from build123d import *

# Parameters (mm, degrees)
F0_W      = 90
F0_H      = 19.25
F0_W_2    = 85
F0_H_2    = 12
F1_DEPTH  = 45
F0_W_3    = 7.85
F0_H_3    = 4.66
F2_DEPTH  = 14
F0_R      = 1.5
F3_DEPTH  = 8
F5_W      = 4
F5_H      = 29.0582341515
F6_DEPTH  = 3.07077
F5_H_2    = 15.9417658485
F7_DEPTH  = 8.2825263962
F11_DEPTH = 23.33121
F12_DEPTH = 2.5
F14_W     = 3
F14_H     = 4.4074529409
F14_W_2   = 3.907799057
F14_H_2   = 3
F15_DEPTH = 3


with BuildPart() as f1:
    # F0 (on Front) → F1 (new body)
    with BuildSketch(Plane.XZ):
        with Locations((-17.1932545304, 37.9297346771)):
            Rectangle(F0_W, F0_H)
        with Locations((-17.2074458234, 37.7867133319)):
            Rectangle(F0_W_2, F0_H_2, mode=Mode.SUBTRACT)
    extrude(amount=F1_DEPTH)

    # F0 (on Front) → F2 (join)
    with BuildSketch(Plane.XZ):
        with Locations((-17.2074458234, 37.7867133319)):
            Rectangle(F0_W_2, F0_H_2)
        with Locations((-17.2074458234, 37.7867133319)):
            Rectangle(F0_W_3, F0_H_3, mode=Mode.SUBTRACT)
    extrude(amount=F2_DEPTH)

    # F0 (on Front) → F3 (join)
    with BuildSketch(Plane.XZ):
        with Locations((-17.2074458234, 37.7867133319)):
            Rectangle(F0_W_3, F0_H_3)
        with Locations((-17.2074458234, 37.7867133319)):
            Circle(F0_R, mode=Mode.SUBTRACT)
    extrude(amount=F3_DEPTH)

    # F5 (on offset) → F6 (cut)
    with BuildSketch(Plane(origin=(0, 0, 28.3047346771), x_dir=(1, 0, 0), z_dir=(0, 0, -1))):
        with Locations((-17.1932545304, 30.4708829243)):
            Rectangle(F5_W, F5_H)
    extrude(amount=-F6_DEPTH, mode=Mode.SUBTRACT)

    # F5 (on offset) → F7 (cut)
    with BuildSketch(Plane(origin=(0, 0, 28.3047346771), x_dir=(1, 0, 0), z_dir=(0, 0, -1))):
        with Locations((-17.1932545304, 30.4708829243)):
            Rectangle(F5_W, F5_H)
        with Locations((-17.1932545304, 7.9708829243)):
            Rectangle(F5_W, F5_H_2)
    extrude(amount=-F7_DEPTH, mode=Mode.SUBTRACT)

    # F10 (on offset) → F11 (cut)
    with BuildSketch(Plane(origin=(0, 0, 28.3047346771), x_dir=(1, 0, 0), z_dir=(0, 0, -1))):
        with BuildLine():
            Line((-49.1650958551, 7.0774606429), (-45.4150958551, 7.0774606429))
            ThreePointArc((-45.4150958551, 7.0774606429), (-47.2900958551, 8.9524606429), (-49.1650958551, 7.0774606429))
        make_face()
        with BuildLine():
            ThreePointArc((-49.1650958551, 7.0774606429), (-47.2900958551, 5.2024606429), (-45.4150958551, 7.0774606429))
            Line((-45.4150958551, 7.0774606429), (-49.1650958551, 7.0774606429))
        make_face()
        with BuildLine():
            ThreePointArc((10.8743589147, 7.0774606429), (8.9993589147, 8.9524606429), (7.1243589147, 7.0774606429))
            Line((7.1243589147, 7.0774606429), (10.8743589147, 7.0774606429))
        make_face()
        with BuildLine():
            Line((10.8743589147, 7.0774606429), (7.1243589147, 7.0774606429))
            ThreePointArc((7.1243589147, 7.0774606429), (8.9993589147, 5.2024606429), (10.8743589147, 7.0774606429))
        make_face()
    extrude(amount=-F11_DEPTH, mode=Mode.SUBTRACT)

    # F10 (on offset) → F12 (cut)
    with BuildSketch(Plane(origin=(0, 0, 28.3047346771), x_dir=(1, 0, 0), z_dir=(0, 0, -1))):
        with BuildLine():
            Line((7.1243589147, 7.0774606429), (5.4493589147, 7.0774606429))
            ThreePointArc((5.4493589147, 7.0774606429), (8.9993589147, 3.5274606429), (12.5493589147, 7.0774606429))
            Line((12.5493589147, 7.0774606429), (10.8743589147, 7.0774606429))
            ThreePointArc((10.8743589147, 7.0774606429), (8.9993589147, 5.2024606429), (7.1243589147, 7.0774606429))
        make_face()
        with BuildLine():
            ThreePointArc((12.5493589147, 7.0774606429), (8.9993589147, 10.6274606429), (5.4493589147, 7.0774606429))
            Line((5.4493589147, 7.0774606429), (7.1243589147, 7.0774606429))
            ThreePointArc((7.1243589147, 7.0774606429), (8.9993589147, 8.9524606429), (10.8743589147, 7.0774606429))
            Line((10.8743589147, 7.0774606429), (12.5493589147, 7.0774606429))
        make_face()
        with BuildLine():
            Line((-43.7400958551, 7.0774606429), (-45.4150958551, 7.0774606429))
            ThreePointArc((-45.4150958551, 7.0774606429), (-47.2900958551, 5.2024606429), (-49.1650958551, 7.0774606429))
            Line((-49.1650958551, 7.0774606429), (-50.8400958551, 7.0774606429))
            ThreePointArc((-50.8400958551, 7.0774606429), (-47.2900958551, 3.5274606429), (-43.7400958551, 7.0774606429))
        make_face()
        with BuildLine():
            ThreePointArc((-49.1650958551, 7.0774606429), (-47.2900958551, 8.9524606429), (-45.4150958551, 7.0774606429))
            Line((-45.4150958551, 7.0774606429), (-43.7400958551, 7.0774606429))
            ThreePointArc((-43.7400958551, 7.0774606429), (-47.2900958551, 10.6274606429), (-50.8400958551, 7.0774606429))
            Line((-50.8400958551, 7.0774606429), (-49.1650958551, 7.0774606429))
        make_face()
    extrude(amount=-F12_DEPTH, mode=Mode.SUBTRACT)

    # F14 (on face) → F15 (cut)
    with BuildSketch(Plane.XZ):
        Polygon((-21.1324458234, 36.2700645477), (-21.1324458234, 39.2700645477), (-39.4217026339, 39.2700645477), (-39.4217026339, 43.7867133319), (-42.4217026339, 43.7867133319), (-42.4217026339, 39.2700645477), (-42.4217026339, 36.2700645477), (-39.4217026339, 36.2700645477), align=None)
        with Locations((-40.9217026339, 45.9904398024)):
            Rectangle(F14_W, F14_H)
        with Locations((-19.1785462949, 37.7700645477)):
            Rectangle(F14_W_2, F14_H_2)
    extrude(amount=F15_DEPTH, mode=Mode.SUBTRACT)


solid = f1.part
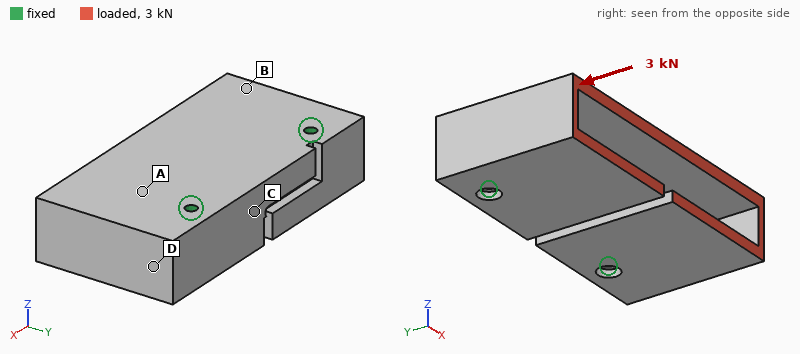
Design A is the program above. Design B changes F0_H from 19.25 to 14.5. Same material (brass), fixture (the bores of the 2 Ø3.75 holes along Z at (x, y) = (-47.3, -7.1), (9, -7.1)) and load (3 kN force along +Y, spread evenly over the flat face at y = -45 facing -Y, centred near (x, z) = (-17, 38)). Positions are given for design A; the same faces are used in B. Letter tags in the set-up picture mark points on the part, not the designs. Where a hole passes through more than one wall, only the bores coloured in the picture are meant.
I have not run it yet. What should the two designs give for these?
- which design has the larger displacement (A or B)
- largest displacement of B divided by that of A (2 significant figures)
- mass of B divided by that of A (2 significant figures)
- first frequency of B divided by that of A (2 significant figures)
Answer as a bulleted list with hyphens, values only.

- B
- 1.4
- 0.58
- 0.41
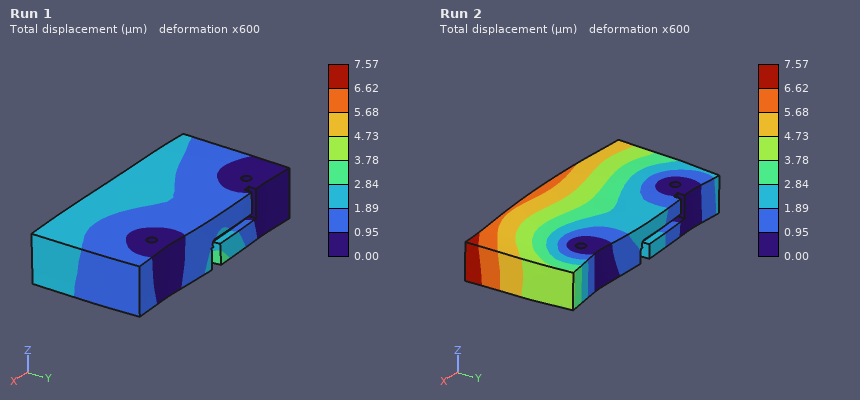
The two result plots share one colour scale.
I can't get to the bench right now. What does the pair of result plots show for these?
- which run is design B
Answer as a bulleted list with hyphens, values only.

- Run 2
